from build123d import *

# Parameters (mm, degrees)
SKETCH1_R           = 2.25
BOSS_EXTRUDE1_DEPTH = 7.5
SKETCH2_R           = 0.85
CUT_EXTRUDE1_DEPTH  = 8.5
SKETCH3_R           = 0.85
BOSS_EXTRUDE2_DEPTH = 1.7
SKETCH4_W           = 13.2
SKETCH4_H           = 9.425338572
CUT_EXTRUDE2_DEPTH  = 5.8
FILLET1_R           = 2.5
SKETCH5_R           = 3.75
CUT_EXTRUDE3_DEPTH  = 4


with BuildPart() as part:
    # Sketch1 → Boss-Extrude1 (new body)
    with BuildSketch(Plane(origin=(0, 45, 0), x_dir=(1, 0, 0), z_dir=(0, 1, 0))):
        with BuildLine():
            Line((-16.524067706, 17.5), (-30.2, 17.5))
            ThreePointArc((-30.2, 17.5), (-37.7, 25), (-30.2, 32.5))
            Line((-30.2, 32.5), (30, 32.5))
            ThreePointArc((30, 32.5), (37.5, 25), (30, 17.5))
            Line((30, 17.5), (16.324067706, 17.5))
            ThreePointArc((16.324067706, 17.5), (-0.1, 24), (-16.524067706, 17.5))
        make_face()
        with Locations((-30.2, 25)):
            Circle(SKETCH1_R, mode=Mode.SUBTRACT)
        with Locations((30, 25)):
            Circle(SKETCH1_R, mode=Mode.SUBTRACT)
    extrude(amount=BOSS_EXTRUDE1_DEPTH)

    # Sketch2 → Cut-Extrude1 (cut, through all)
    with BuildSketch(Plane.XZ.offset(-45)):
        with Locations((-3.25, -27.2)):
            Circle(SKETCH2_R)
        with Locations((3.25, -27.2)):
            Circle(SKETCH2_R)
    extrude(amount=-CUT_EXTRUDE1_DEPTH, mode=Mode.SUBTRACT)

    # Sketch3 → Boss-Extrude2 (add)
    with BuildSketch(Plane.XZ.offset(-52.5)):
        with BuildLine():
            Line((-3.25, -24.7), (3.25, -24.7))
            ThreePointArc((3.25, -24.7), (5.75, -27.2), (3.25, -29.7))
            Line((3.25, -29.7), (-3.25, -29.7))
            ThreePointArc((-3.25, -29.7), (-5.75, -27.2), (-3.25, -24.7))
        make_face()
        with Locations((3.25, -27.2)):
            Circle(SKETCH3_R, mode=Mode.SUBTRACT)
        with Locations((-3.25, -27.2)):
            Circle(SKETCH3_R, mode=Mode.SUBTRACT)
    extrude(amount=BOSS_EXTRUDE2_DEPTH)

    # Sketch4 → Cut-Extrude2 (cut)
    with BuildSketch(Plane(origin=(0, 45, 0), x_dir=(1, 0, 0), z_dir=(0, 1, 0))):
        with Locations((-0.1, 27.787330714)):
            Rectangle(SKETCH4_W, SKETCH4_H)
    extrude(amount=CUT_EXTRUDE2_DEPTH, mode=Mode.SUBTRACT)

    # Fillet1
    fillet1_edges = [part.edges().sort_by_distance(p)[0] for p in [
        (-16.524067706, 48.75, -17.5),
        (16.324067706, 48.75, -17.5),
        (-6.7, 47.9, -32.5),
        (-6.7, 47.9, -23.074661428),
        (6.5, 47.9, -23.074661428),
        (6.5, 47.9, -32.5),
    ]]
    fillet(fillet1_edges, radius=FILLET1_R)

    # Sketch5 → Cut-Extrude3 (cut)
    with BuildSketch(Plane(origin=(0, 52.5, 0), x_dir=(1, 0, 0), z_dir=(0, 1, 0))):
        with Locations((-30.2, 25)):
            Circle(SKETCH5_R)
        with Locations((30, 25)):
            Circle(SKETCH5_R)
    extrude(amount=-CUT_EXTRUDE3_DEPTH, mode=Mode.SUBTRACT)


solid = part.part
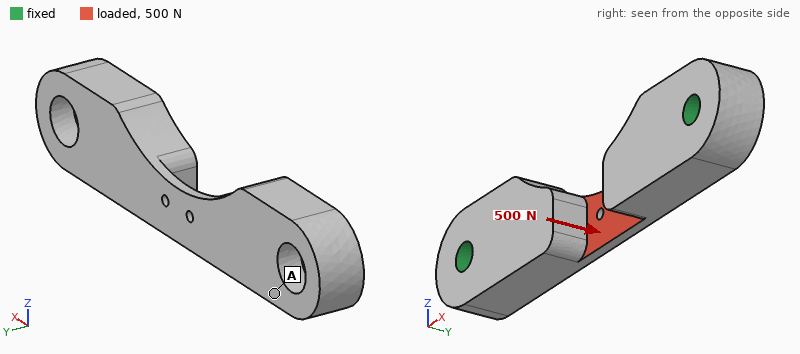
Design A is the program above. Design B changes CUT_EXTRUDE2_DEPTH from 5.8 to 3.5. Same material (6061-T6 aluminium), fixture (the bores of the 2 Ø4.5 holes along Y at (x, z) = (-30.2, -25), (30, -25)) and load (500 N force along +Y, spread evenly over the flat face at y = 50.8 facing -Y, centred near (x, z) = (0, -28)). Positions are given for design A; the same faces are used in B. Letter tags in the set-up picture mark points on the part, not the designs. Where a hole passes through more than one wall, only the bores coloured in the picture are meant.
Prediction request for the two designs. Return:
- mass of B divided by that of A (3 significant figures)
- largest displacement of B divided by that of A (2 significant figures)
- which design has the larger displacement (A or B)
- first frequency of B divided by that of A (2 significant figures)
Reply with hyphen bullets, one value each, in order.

- 1.05
- 0.69
- A
- 0.94
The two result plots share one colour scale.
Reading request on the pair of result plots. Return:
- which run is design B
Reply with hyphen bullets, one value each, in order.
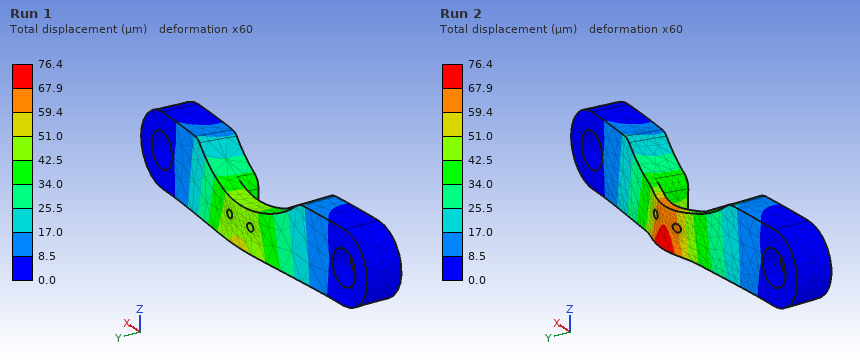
- Run 1
